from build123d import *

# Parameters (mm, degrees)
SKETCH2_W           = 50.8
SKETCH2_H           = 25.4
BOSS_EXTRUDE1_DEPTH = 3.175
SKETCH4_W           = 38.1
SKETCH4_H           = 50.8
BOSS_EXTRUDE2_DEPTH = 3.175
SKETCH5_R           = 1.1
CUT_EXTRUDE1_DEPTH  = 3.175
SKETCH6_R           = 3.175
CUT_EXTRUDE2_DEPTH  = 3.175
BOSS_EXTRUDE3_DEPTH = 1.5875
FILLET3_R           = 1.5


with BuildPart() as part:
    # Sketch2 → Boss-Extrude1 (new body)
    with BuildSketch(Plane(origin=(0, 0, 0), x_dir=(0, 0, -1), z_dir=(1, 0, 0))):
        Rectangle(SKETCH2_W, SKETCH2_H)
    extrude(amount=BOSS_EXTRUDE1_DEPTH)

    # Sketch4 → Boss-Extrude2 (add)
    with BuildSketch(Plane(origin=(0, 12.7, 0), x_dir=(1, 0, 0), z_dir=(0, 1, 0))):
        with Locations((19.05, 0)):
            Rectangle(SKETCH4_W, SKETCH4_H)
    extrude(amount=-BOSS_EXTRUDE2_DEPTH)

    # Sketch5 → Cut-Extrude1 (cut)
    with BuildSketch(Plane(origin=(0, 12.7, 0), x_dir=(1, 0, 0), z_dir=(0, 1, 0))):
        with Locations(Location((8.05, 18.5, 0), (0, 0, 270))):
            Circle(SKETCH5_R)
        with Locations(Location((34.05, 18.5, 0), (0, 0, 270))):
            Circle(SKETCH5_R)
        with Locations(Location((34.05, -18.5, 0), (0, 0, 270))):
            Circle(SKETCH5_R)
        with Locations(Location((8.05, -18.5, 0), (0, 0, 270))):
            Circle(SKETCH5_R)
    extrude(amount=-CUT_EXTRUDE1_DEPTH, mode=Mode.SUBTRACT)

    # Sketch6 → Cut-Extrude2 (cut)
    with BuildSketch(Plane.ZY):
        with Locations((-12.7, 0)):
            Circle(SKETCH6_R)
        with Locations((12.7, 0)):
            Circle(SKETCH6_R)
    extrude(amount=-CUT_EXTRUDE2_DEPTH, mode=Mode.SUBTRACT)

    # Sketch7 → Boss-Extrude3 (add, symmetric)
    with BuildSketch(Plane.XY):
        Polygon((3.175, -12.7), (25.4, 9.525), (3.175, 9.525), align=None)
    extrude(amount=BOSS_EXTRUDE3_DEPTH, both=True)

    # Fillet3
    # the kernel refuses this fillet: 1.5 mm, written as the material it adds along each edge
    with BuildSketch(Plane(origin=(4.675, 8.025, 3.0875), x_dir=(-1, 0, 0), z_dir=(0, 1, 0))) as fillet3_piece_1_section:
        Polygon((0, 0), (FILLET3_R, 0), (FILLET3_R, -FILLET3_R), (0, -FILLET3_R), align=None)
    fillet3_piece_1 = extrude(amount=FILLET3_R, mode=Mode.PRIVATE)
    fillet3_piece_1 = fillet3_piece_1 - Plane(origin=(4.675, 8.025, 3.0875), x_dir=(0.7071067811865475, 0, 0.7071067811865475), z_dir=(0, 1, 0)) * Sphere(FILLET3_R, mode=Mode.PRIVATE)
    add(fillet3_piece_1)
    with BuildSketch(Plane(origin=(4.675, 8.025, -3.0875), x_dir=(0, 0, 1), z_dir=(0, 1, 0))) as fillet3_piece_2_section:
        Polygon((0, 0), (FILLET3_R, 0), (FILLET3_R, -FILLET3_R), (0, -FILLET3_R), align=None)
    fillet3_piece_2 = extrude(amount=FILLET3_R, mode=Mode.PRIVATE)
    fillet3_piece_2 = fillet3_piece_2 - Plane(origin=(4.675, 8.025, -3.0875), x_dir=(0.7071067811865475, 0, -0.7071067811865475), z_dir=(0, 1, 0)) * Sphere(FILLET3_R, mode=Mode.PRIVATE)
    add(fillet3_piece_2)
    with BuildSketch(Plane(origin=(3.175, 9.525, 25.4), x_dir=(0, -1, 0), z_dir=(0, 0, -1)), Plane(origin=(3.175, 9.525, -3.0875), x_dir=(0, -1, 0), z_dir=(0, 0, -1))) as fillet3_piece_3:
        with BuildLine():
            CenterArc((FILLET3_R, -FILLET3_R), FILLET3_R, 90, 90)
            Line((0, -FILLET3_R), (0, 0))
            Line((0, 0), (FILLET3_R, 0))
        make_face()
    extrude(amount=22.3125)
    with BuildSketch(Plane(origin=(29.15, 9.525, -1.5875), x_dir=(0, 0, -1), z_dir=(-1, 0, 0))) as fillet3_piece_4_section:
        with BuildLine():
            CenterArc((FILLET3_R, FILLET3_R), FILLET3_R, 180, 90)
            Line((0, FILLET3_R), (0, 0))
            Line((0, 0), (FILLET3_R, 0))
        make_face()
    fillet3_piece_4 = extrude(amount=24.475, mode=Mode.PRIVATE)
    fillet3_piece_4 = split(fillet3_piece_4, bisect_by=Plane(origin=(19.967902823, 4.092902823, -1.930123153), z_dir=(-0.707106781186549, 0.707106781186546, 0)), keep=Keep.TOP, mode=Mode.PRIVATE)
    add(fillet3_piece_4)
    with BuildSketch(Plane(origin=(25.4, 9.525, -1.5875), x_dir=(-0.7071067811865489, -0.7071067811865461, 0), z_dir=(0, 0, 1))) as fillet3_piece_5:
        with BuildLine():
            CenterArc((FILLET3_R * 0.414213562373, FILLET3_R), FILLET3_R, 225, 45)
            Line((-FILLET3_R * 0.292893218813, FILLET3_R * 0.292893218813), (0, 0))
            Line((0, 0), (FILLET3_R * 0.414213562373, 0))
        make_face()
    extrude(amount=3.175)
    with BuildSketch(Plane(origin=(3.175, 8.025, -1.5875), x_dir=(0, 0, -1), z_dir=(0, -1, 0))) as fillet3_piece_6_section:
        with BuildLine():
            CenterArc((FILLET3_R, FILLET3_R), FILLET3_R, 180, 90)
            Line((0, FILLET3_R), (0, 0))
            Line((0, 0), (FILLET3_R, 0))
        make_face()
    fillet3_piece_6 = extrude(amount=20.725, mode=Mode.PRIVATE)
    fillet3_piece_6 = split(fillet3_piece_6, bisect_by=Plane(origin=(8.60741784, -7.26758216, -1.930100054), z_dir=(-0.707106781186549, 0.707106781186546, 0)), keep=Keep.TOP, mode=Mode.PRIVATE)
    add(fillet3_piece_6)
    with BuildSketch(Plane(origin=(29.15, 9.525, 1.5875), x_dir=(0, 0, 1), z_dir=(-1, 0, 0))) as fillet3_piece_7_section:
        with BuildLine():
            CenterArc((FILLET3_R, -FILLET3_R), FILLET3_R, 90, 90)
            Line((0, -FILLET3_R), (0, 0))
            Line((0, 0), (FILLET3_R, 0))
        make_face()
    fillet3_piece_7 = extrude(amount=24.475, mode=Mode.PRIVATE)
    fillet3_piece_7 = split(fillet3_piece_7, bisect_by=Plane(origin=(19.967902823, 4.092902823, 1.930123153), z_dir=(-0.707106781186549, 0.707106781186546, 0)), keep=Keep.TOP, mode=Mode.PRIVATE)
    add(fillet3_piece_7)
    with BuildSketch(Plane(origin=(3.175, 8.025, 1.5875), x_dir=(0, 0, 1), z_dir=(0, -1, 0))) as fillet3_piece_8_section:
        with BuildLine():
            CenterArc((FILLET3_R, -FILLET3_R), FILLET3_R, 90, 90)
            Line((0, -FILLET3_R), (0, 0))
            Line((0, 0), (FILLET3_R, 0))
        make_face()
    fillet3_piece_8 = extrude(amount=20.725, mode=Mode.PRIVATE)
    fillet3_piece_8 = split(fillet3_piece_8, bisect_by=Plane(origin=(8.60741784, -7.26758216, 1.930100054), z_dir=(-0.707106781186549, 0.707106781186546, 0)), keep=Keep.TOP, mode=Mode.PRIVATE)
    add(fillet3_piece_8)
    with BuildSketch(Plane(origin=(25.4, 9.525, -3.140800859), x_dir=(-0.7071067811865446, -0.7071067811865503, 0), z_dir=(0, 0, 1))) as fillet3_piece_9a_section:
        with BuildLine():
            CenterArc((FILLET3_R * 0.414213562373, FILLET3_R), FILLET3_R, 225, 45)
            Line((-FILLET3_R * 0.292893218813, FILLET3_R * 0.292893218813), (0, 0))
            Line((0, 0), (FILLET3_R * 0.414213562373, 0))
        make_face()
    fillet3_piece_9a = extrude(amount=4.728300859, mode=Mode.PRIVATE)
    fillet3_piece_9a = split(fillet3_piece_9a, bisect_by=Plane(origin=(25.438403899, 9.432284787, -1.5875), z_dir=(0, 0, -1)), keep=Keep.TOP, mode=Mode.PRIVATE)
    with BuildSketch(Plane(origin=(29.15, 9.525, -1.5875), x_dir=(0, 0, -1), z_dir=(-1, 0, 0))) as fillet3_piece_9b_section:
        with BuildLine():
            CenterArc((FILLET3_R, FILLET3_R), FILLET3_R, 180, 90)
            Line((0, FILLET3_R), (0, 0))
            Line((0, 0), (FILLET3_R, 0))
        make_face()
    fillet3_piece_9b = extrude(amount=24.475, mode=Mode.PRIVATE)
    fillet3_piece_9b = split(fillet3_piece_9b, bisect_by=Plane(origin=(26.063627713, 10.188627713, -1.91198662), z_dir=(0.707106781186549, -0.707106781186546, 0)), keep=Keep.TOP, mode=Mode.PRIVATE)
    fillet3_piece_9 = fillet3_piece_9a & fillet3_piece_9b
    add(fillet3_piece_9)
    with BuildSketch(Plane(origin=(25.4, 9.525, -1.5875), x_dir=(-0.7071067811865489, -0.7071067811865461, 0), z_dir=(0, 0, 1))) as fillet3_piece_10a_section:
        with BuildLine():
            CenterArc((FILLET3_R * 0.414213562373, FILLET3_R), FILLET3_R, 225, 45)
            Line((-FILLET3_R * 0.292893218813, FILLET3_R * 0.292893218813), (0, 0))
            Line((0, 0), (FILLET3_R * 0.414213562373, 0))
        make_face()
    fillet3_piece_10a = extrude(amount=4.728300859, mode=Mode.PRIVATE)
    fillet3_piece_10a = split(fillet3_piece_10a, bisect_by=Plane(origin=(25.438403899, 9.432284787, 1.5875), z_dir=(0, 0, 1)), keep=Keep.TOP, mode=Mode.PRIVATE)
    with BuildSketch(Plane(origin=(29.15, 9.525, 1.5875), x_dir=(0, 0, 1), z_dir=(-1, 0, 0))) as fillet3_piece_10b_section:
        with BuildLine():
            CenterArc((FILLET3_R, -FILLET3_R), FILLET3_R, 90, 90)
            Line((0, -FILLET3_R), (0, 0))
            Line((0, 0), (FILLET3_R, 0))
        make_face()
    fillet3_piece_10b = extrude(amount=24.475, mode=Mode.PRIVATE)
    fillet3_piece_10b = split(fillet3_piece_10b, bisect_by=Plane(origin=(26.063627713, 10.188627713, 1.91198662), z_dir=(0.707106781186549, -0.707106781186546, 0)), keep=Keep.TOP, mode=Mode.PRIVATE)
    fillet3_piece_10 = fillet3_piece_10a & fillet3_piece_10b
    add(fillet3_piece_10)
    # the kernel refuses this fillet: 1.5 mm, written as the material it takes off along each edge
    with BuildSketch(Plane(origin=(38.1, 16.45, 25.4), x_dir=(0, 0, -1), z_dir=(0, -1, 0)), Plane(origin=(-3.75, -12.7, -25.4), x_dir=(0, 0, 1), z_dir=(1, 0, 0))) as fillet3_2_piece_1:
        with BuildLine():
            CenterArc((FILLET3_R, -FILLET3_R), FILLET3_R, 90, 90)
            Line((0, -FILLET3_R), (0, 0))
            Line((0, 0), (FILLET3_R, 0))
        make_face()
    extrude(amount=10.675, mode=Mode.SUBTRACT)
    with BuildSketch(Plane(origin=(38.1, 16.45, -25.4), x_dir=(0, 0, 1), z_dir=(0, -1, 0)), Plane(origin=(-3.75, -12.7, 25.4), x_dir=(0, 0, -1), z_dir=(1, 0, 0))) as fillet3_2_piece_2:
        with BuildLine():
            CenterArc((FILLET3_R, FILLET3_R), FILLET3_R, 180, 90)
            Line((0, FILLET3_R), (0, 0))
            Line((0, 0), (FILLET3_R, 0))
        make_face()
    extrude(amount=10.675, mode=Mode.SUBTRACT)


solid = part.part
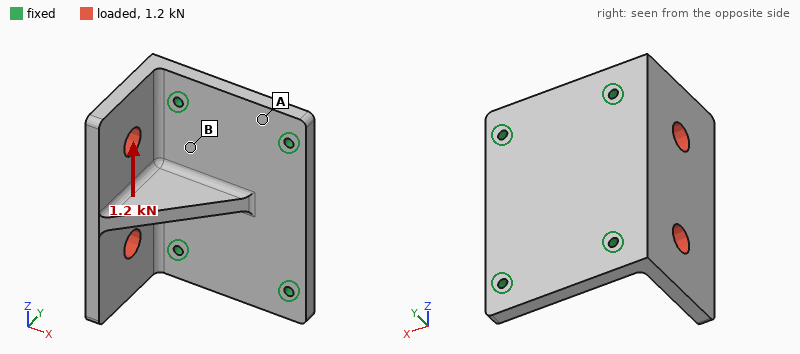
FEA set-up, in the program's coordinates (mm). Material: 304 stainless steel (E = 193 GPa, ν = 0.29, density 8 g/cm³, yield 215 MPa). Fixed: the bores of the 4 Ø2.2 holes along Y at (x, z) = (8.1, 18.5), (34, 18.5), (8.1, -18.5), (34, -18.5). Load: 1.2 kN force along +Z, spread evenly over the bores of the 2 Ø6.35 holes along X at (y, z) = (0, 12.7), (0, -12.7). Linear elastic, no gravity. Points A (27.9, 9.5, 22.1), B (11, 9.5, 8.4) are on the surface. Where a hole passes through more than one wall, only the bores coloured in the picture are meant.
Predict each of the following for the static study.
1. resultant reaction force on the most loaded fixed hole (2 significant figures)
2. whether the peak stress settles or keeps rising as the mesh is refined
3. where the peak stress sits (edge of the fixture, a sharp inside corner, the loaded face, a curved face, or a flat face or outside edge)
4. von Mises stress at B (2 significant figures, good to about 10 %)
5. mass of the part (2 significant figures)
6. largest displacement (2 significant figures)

690 N
keeps rising
edge of the fixture
12 MPa
83 g
11 µm
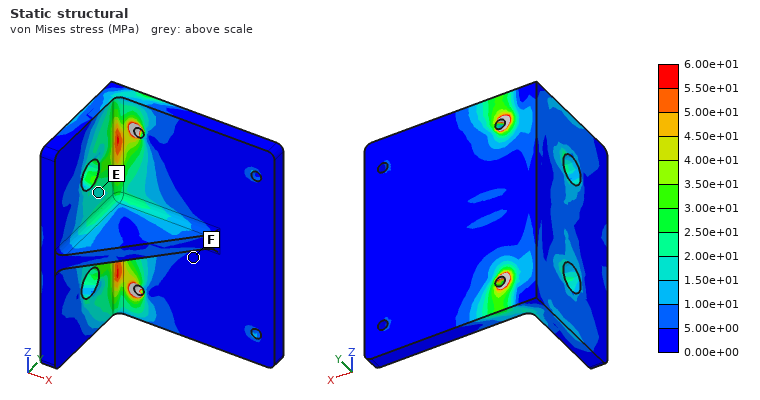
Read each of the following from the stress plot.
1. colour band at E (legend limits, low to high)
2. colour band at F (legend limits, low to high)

1.50e+01 to 2.00e+01 MPa
0.00e+00 to 5.00e+00 MPa
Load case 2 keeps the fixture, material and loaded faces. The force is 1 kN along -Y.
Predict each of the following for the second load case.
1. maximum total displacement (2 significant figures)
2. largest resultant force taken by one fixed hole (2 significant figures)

19 µm
570 N
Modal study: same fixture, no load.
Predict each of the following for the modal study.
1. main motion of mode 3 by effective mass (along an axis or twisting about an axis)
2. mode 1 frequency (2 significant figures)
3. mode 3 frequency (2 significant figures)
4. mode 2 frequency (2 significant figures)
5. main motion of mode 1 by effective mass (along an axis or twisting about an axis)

along Y
4900 Hz
9400 Hz
5900 Hz
along X
